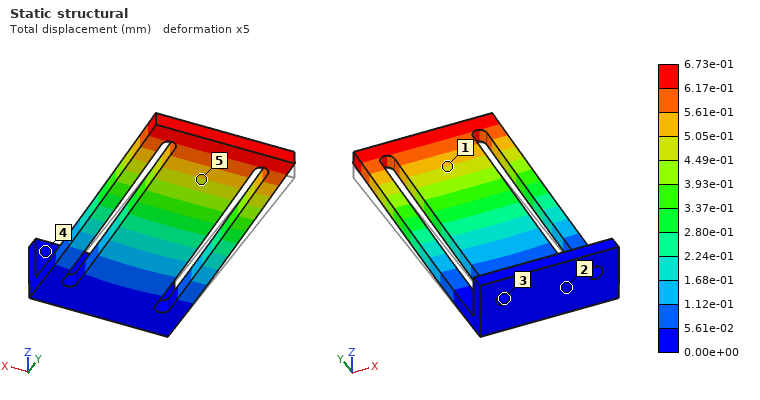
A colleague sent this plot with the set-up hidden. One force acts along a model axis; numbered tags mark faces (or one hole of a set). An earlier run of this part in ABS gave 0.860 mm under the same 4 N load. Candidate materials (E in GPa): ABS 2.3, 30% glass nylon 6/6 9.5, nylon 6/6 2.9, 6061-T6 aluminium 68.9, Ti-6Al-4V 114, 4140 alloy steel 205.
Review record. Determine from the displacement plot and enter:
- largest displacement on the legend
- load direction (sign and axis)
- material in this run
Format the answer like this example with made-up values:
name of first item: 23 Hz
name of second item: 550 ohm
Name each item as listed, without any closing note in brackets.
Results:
largest displacement on the legend: 6.73e-01 mm
load direction: +Z
material in this run: nylon 6/6
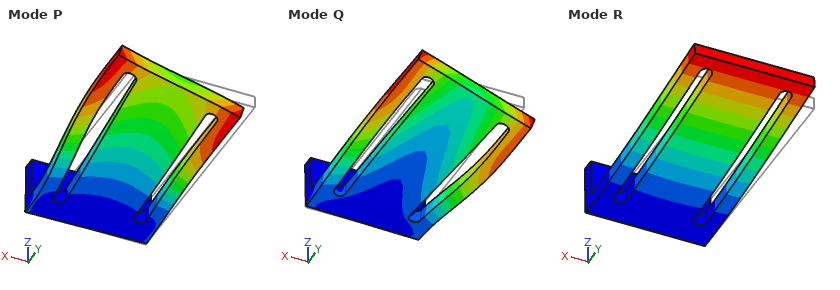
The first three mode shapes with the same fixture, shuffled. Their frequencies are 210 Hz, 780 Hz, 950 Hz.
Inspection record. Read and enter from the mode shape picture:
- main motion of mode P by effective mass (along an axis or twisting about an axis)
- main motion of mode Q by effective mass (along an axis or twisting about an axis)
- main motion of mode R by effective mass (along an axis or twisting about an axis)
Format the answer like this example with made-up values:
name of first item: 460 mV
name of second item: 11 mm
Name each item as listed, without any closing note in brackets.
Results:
main motion of mode P by effective mass: along X
main motion of mode Q by effective mass: along X
main motion of mode R by effective mass: along Z
